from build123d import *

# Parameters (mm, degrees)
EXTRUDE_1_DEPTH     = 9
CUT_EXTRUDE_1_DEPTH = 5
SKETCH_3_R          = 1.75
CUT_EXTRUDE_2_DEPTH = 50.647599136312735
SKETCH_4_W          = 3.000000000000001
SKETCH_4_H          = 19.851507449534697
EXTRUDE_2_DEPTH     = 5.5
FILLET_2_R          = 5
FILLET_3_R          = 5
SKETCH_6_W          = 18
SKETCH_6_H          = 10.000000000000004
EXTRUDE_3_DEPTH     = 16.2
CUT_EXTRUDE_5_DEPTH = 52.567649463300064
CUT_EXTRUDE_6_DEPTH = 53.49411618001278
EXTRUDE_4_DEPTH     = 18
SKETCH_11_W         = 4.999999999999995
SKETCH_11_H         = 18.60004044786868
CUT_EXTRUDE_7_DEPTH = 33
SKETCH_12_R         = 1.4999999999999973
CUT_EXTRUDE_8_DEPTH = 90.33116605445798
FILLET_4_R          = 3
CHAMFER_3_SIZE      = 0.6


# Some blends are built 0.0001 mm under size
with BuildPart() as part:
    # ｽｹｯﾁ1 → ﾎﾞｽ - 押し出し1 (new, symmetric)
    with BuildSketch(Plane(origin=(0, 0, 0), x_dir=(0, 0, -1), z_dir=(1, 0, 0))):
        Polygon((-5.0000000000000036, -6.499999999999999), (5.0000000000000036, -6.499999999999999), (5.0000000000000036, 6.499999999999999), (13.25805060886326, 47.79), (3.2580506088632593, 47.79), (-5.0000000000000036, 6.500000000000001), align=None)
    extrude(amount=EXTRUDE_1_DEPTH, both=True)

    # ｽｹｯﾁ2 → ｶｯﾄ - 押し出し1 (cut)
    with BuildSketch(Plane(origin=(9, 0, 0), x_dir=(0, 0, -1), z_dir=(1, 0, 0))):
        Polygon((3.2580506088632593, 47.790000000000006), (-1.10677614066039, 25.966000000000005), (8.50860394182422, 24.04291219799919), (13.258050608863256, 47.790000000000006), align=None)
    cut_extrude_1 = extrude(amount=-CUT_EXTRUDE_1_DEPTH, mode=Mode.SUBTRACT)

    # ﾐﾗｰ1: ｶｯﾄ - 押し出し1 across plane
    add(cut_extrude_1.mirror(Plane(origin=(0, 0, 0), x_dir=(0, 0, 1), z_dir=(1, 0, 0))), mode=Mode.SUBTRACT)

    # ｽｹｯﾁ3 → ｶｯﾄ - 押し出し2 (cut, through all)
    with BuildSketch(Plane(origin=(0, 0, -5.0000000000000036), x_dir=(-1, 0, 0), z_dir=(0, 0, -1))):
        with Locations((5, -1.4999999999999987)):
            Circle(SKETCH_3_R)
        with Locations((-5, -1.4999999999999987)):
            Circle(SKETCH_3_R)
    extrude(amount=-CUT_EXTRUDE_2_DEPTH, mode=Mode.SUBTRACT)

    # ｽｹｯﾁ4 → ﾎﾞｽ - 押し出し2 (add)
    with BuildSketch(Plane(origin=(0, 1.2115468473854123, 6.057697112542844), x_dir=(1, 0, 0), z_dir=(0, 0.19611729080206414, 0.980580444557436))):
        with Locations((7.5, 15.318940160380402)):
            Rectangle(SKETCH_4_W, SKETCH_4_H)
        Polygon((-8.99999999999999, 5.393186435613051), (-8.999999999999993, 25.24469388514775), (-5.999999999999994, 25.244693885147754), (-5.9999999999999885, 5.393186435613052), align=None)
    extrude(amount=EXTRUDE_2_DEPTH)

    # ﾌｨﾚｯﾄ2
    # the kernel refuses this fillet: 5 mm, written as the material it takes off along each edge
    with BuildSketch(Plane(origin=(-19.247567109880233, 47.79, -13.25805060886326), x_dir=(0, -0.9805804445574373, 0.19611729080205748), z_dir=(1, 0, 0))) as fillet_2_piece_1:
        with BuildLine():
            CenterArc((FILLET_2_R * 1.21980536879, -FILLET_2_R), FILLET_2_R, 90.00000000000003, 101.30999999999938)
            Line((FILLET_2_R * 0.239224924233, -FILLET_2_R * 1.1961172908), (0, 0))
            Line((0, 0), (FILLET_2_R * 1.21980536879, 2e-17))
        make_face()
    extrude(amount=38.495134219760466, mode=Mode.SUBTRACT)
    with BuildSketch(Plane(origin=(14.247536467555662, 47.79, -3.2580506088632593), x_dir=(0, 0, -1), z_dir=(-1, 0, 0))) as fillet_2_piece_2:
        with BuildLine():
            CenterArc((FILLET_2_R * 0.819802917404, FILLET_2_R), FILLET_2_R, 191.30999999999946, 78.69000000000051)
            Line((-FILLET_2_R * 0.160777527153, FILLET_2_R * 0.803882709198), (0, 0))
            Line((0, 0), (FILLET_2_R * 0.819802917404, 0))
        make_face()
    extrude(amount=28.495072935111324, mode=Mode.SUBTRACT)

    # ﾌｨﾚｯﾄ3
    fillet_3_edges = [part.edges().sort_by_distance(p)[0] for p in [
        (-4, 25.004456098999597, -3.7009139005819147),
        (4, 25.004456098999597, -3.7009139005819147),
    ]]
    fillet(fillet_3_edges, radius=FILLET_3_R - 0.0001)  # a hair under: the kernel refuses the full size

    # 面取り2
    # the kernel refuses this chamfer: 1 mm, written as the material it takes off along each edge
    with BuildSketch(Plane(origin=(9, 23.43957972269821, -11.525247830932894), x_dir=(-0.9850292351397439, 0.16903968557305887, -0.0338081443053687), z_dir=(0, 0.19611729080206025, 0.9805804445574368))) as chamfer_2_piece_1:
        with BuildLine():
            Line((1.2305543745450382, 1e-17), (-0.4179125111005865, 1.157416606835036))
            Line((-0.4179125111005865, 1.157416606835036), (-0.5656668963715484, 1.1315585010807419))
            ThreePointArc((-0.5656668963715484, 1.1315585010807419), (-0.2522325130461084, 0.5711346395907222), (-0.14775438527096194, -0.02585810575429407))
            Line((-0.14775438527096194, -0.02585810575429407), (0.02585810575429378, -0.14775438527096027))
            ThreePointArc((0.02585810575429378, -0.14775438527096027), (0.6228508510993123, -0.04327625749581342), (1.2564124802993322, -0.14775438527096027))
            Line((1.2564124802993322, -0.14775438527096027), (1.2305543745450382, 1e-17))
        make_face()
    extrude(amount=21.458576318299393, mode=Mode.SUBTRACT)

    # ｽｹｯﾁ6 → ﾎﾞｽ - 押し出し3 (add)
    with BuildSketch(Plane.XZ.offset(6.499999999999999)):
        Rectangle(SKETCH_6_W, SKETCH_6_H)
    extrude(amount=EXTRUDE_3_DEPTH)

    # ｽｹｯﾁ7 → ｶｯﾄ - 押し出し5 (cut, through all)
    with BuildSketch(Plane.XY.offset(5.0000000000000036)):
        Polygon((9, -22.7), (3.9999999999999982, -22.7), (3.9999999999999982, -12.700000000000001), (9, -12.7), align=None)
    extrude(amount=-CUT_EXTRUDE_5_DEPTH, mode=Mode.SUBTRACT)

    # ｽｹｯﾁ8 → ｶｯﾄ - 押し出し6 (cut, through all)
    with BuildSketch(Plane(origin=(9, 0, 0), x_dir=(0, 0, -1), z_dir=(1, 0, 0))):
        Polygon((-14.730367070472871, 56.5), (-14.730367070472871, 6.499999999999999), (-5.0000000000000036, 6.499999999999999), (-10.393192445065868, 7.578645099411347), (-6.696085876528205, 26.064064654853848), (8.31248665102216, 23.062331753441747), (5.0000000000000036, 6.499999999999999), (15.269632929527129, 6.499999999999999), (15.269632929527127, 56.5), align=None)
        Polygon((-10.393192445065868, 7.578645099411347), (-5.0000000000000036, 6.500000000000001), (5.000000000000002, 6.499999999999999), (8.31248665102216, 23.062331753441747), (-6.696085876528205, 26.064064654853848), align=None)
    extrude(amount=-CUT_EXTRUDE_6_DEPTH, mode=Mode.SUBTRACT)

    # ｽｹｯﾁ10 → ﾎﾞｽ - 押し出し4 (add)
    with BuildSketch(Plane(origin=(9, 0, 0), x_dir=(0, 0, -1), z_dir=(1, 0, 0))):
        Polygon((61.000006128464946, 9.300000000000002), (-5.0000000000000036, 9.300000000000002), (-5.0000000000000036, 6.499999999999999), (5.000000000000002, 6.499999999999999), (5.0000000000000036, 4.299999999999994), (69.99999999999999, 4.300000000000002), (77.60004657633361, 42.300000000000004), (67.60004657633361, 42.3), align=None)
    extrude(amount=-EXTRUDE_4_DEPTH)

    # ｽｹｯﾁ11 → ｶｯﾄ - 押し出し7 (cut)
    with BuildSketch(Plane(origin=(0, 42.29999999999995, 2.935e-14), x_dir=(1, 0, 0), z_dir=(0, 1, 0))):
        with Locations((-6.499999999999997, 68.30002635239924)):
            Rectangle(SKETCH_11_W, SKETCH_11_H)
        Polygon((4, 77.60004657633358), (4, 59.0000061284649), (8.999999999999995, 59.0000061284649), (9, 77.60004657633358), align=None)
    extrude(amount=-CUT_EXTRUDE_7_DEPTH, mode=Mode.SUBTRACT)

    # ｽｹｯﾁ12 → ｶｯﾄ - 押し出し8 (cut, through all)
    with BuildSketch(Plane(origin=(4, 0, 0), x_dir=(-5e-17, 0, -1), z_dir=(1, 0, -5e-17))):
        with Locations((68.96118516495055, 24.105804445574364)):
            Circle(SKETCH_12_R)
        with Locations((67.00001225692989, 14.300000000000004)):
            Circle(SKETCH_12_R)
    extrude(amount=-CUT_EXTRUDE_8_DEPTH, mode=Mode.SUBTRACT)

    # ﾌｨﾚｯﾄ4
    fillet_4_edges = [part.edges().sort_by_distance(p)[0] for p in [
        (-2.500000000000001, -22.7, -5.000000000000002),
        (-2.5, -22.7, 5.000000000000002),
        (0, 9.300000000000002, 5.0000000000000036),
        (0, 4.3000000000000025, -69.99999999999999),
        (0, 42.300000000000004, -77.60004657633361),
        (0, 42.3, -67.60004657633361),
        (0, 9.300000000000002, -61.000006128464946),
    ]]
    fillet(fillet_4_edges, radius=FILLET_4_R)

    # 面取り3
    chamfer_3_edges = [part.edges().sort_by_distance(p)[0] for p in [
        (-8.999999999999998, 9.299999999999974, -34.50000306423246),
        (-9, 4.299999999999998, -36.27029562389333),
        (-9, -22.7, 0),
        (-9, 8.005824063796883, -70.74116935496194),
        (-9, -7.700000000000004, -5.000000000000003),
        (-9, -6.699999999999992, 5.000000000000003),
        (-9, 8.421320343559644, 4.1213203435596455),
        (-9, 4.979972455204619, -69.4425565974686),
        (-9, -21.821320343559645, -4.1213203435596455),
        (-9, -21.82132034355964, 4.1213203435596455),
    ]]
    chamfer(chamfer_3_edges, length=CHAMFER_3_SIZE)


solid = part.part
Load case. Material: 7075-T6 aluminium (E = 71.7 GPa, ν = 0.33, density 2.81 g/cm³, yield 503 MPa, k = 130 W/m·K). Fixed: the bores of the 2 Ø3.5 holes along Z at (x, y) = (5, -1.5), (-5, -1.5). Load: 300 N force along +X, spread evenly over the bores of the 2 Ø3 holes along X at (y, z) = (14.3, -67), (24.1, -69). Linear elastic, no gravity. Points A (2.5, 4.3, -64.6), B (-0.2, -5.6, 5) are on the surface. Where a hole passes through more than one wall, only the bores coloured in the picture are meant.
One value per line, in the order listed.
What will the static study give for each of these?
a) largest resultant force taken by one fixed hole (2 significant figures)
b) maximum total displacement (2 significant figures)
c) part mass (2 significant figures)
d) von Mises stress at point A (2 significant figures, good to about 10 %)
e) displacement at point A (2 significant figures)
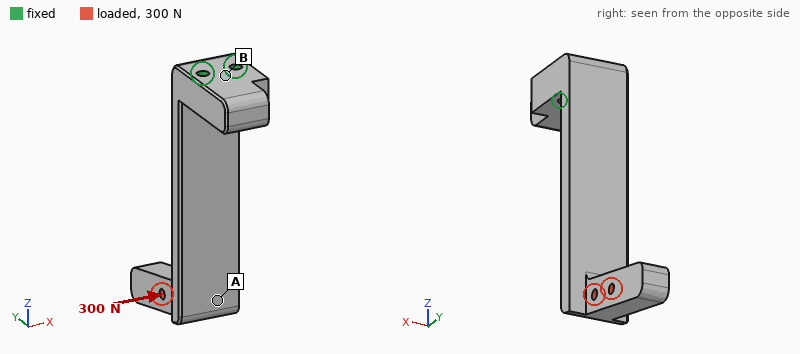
1.4 kN
0.71 mm
37 g
22 MPa
0.19 mm
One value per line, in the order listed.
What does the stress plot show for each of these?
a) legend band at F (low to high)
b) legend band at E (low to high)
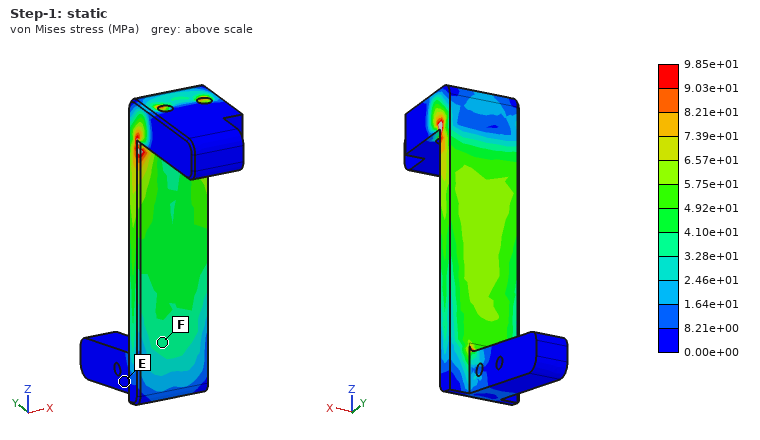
3.28e+01 to 4.10e+01 MPa
0.00e+00 to 8.21e+00 MPa
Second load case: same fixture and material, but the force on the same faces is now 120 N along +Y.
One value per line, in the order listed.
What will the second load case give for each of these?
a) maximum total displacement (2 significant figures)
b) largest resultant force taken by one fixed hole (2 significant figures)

1.2 mm
150 N
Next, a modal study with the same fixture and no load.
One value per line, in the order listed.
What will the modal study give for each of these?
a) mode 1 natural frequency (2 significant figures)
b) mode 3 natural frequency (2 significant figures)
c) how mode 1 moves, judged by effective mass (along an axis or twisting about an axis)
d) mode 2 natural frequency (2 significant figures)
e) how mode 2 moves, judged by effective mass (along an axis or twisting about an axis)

510 Hz
2400 Hz
along Y
1200 Hz
along X
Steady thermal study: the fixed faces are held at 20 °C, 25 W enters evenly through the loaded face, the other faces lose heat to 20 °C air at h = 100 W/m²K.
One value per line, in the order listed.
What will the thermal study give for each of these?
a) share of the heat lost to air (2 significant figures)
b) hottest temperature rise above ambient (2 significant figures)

69 %
75 K
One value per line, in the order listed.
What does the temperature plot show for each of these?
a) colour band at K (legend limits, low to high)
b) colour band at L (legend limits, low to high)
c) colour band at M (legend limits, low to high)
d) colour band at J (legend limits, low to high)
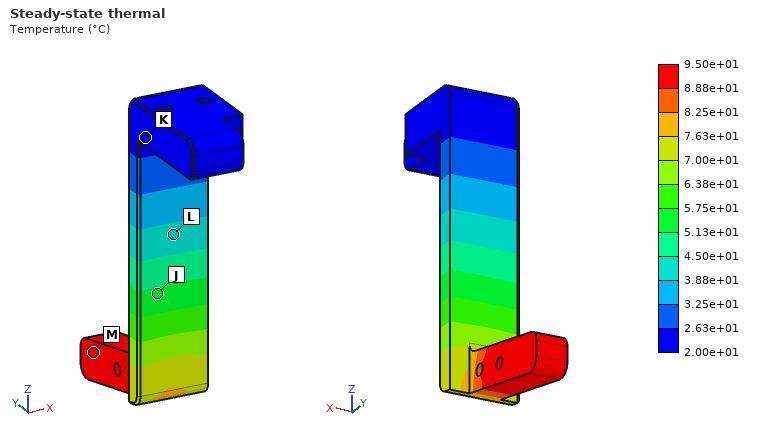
2.00e+01 to 2.63e+01 °C
3.88e+01 to 4.50e+01 °C
8.88e+01 to 9.50e+01 °C
5.13e+01 to 5.75e+01 °C
